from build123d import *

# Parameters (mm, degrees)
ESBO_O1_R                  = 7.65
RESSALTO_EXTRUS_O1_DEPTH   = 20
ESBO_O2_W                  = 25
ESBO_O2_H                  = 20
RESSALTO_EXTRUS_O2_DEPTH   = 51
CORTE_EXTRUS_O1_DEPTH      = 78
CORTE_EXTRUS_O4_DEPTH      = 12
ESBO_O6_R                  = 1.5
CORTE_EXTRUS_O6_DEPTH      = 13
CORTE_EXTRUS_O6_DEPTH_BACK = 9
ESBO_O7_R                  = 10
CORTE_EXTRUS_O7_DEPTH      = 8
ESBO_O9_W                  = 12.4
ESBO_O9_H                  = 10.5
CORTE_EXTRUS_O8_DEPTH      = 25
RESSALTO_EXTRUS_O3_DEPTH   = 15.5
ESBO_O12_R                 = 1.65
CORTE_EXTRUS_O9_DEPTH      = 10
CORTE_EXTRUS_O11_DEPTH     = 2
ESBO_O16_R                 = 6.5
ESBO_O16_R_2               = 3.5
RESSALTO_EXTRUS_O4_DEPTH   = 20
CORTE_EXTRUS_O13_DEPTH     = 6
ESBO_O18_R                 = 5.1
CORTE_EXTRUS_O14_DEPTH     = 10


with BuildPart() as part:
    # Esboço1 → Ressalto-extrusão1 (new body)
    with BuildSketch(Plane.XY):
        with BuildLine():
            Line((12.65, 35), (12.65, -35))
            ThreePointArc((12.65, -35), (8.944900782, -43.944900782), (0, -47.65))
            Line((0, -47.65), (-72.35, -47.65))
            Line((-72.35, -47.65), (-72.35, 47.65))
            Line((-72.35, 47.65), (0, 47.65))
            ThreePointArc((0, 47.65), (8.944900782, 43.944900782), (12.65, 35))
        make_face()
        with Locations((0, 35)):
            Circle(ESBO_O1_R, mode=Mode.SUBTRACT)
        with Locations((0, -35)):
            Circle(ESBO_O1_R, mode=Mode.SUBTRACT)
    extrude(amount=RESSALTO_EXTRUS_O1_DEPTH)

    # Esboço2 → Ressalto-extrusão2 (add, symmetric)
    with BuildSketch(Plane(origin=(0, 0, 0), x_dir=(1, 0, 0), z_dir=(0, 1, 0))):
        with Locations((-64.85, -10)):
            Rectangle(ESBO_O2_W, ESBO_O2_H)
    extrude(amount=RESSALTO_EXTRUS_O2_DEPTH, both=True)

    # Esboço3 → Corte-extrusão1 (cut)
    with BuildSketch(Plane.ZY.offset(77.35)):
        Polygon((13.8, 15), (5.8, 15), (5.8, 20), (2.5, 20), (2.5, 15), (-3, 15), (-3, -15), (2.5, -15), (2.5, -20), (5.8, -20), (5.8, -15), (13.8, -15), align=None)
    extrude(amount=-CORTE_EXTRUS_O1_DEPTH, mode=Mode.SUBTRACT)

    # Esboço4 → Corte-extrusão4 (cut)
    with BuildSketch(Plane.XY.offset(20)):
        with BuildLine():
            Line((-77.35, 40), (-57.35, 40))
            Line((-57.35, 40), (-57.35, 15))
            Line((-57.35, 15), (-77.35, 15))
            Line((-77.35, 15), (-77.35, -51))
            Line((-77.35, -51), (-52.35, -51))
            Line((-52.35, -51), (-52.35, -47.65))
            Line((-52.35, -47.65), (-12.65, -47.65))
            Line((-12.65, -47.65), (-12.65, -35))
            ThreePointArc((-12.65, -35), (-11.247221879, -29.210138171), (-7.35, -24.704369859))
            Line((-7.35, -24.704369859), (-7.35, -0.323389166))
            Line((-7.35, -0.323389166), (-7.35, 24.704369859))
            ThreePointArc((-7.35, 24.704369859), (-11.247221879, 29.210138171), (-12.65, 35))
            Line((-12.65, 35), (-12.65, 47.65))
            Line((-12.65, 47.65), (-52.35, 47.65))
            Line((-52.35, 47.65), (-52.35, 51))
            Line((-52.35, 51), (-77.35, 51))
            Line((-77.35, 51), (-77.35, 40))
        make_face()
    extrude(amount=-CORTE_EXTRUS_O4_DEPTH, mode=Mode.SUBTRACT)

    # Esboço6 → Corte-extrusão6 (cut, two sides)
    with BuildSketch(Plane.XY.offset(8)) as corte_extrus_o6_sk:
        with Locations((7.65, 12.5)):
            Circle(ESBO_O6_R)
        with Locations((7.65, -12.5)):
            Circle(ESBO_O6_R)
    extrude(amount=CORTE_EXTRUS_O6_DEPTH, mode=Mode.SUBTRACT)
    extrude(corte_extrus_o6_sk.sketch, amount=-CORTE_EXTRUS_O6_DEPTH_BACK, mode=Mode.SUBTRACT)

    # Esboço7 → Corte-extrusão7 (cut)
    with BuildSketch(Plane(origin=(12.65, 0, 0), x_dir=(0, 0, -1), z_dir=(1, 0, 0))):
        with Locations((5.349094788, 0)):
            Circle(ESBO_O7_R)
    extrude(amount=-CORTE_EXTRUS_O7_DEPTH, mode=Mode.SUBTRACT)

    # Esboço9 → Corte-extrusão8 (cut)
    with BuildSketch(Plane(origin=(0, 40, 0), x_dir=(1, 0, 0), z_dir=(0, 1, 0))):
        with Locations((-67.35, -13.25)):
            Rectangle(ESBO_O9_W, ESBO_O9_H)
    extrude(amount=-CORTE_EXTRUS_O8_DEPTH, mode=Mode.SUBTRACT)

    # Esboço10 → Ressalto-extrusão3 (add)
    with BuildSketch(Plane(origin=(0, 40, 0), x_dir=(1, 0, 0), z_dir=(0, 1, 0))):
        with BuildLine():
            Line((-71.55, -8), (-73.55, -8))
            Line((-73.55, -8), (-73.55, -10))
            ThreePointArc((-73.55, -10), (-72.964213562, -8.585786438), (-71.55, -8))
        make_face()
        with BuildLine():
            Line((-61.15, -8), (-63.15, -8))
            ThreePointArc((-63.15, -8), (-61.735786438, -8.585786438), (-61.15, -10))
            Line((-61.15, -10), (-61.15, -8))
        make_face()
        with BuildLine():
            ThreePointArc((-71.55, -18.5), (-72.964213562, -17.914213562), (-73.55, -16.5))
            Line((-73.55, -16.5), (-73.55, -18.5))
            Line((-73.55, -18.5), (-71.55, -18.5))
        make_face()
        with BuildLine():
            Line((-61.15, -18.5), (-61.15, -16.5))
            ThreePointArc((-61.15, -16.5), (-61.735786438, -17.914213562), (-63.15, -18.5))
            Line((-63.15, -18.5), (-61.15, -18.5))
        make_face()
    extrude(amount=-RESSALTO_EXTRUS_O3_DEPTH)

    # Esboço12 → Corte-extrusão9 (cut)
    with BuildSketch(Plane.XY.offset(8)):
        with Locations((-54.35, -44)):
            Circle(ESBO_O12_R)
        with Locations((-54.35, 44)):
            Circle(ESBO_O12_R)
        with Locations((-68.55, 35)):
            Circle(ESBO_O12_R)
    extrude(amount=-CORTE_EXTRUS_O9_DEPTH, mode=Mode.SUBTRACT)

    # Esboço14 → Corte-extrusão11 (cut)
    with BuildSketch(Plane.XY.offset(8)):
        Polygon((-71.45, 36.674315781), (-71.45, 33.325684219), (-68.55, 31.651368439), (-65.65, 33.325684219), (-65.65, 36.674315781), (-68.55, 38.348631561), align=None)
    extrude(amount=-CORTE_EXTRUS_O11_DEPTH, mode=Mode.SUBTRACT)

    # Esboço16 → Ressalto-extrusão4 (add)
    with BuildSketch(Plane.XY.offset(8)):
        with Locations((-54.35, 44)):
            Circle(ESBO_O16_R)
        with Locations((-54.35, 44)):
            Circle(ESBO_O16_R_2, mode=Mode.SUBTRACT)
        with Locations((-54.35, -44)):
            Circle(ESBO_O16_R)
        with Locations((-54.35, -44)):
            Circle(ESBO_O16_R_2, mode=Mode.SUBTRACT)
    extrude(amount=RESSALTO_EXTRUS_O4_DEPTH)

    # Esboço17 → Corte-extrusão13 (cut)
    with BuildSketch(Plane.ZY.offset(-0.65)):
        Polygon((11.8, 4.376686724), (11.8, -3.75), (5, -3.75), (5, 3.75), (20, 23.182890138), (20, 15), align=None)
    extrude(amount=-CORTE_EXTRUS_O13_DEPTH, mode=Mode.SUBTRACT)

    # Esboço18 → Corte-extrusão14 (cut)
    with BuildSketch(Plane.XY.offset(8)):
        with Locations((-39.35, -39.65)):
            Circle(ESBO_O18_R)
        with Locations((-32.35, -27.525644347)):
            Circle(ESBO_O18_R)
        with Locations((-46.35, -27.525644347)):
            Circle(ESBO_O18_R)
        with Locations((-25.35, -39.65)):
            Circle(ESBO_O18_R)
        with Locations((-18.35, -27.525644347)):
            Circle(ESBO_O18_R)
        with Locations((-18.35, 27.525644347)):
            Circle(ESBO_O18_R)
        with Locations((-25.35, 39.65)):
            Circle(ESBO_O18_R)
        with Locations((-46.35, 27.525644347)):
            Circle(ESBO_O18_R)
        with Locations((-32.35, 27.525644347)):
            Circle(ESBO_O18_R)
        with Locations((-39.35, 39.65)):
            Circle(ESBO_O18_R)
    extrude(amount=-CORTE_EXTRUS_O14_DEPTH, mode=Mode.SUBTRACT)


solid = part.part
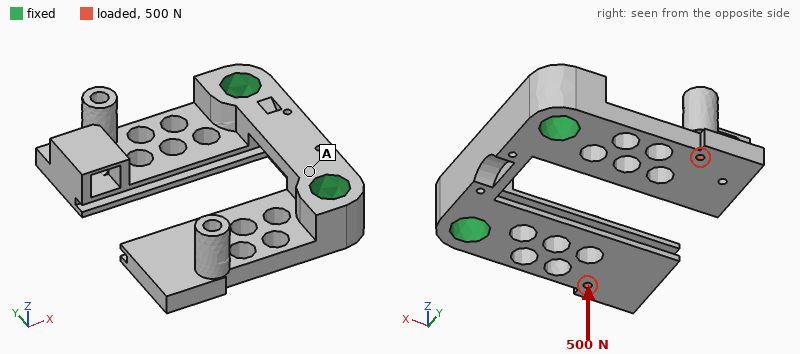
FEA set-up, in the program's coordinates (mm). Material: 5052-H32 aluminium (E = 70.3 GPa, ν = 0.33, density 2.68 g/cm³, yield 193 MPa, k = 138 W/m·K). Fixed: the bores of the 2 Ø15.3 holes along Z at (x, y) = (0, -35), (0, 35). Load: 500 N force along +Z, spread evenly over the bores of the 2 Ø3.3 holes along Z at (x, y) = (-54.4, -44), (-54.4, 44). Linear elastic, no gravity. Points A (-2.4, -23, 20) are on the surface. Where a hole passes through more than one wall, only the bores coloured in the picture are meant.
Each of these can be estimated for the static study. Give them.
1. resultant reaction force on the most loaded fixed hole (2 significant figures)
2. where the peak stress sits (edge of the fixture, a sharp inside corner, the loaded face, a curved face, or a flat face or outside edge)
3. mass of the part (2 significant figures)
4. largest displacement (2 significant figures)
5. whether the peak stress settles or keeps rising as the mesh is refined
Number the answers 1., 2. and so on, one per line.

1. 250 N
2. a sharp inside corner
3. 170 g
4. 0.30 mm
5. keeps rising
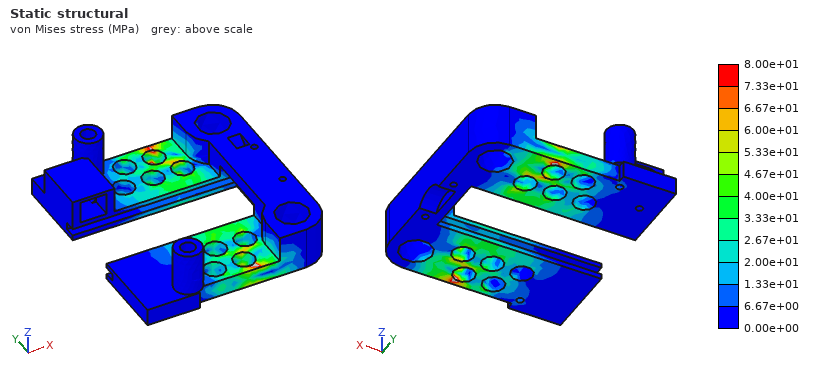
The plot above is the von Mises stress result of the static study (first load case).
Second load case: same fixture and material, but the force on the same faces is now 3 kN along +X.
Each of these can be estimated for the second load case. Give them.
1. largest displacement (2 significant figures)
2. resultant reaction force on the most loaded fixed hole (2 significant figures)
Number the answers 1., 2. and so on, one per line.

1. 55 µm
2. 1.5 kN
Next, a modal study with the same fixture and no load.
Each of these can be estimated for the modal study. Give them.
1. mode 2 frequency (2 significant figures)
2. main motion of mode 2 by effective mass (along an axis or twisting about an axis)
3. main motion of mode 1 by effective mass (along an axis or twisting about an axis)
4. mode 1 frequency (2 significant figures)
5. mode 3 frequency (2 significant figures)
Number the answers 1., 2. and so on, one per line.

1. 960 Hz
2. along Z
3. along Z
4. 820 Hz
5. 2100 Hz
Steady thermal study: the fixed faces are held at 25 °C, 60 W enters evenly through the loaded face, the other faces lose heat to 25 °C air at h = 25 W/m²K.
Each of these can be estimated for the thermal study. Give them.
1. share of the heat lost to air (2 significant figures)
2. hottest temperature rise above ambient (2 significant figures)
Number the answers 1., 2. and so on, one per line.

1. 32 %
2. 67 K
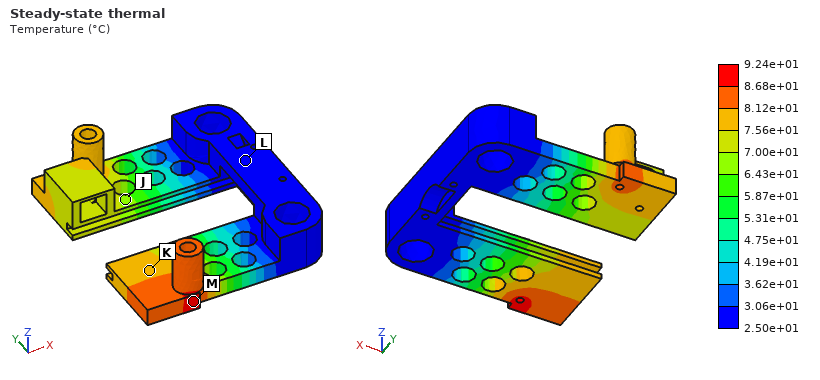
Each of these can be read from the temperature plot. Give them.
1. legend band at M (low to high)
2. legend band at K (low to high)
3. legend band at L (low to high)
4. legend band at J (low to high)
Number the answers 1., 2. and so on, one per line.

1. 8.68e+01 to 9.24e+01 °C
2. 7.56e+01 to 8.12e+01 °C
3. 2.50e+01 to 3.06e+01 °C
4. 6.43e+01 to 7.00e+01 °C
